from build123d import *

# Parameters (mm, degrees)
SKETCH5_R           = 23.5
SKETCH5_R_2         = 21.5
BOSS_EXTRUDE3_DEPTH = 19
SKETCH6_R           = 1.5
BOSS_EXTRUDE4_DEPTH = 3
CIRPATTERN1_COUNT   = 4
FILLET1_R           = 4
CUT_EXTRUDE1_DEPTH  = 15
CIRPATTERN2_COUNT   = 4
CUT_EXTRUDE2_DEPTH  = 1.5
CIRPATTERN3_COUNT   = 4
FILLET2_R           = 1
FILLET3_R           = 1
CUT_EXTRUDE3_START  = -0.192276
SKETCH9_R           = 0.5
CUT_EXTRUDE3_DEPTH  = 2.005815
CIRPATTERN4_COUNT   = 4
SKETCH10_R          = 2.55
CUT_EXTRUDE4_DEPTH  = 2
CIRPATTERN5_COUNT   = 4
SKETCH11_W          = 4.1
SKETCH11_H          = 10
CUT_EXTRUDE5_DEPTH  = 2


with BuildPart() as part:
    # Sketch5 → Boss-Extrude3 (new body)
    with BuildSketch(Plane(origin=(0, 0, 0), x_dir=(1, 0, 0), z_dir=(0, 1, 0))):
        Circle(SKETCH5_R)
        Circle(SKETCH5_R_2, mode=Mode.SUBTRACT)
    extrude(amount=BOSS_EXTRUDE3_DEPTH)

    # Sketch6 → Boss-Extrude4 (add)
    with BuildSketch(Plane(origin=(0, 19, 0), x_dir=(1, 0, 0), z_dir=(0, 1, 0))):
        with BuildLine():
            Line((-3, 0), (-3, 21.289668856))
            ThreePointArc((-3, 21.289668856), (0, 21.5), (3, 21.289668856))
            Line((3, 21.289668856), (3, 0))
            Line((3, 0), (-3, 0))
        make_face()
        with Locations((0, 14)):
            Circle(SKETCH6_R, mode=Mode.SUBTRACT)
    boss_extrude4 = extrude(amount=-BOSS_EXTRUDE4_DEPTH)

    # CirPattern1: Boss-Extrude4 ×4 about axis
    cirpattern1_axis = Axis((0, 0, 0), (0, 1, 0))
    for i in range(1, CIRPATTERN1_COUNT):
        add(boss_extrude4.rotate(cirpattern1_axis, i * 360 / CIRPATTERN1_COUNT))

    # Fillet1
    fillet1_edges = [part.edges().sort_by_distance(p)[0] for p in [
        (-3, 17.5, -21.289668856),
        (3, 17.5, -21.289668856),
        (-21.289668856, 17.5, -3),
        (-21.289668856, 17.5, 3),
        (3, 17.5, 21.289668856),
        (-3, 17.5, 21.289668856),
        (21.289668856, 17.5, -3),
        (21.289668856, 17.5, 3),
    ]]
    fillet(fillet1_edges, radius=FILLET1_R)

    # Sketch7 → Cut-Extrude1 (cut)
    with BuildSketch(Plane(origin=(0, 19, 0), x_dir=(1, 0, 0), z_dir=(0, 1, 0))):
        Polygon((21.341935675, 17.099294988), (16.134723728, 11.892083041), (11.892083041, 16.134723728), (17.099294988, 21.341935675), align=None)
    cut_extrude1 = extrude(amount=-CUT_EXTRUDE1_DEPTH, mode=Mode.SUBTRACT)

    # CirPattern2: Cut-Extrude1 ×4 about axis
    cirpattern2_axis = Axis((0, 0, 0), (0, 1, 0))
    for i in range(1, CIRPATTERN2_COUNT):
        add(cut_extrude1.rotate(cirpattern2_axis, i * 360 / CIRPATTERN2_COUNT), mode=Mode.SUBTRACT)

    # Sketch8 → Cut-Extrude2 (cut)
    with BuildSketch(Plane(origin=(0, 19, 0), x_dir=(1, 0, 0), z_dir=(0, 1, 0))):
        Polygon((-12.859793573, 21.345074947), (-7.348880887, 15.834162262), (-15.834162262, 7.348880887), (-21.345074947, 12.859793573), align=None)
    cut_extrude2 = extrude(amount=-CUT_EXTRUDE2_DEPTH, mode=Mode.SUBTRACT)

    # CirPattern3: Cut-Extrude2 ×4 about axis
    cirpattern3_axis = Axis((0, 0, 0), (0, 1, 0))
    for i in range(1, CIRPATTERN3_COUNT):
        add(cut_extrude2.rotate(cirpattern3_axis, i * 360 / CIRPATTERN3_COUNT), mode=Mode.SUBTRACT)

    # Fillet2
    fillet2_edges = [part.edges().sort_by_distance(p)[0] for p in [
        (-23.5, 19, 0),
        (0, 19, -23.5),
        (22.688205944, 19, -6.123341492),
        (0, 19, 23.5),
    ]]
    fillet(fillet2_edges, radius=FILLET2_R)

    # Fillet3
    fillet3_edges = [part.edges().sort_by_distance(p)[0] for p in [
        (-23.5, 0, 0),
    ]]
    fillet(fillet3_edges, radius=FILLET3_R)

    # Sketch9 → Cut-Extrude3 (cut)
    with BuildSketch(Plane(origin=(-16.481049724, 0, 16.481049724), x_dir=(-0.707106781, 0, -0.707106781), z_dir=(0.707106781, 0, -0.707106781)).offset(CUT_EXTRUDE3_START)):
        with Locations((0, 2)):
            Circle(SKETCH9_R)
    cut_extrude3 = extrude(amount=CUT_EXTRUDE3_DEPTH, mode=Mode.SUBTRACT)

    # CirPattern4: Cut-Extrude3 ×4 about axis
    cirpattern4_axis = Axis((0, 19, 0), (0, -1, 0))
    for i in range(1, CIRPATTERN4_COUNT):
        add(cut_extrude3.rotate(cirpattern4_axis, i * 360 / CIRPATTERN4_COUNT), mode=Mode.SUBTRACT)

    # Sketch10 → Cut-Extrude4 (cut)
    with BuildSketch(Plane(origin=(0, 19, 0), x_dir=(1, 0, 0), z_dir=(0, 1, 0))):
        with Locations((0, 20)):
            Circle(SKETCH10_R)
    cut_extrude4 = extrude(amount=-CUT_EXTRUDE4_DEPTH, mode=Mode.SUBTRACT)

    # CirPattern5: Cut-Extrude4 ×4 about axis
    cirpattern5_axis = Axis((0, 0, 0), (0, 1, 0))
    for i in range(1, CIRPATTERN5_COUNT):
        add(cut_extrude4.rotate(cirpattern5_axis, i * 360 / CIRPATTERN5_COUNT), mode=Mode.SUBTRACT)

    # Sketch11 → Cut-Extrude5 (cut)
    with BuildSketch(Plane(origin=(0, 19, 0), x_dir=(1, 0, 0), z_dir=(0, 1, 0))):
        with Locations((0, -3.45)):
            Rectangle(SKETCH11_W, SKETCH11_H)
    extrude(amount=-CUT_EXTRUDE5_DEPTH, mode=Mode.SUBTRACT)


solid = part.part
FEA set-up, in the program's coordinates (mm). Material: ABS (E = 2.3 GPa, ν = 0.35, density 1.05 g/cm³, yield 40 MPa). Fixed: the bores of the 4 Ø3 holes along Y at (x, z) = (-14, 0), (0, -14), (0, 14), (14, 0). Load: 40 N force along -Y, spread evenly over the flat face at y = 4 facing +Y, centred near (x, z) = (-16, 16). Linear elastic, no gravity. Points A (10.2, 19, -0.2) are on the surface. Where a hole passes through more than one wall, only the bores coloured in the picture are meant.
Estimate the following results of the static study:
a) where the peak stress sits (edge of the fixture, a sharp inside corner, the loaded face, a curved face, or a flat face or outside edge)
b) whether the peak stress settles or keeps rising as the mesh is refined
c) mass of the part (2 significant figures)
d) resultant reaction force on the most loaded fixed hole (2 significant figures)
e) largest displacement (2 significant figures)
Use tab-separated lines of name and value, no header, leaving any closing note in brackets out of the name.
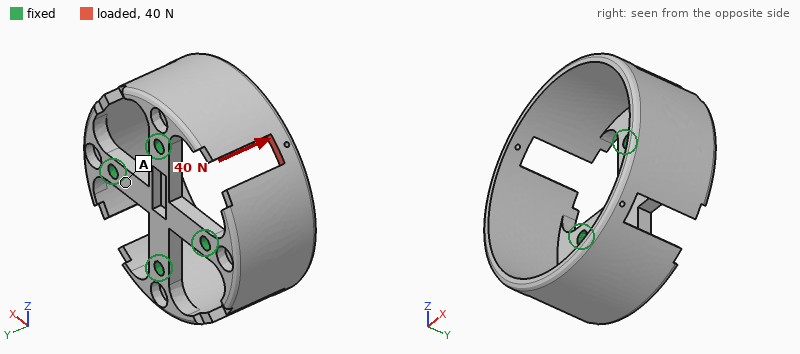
where the peak stress sits	a sharp inside corner
whether the peak stress settles or keeps rising as the mesh is refined	keeps rising
mass of the part	6.1 g
resultant reaction force on the most loaded fixed hole	27 N
largest displacement	0.48 mm
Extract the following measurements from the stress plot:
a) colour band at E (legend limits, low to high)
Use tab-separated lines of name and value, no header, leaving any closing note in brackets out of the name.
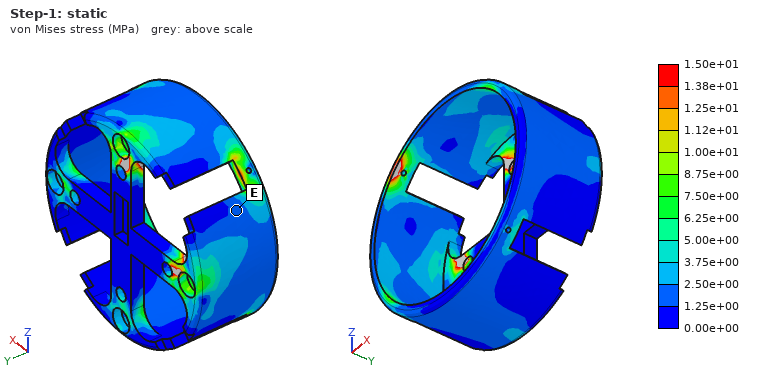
colour band at E	1.25e+00 to 2.50e+00 MPa
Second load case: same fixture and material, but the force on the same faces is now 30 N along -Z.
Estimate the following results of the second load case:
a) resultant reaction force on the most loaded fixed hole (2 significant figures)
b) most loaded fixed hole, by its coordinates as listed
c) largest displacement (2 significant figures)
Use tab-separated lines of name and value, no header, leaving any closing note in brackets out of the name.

resultant reaction force on the most loaded fixed hole	22 N
most loaded fixed hole, by its coordinates as listed	(-14, 0)
largest displacement	0.54 mm
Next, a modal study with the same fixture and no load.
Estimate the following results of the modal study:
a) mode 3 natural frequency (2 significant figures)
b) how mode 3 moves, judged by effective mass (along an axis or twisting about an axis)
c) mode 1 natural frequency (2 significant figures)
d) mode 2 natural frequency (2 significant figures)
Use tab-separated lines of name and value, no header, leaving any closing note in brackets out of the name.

mode 3 natural frequency	1600 Hz
how mode 3 moves, judged by effective mass	along X
mode 1 natural frequency	1100 Hz
mode 2 natural frequency	1400 Hz
